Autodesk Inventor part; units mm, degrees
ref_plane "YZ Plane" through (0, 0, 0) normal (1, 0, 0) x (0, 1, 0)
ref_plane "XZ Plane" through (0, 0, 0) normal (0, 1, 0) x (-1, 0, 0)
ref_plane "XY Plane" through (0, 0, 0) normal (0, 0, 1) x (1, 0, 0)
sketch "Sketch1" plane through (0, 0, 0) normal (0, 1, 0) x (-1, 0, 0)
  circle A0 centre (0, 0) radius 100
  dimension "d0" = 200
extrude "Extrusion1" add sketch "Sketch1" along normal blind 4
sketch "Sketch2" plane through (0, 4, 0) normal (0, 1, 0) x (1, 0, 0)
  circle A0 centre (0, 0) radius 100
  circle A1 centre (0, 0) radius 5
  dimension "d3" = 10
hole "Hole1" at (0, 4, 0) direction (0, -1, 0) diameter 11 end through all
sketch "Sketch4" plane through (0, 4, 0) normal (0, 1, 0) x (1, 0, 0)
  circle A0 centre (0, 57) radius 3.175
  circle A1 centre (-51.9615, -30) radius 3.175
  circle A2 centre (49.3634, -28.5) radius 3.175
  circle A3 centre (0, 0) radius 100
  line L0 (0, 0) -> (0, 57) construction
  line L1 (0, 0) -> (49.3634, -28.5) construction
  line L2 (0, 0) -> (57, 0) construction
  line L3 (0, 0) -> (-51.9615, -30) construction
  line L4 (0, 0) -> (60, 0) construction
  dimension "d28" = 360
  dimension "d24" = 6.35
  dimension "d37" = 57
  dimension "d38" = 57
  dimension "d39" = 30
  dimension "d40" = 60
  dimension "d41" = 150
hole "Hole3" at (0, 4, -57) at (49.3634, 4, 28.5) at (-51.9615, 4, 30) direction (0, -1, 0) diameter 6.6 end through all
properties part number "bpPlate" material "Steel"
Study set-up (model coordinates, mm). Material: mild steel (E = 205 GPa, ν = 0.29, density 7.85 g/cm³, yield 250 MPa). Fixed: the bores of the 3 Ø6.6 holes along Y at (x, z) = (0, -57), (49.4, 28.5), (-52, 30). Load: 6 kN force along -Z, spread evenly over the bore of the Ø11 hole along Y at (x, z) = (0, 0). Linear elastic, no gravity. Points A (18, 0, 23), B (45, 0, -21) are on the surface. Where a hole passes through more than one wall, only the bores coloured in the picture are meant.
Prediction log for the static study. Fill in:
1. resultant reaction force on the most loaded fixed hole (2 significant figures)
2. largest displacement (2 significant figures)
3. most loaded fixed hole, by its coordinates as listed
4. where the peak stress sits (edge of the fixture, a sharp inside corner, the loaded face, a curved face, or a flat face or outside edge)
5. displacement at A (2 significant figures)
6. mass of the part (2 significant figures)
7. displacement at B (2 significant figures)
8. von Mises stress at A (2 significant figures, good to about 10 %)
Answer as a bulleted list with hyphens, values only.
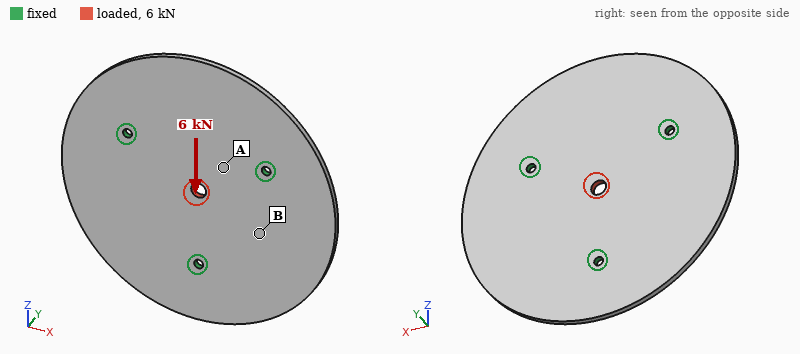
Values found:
- 2.3 kN
- 6.4 µm
- (0, -57)
- the loaded face
- 3.1 µm
- 980 g
- 1.7 µm
- 12 MPa
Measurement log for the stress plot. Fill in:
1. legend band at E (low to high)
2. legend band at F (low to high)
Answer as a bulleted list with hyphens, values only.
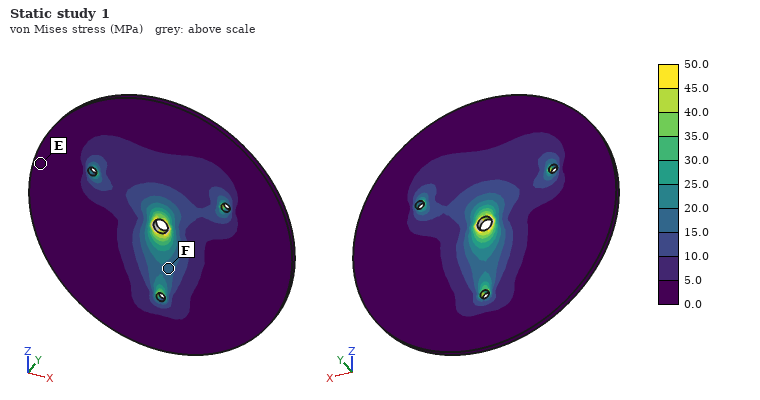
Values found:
- 0.0 to 5.0 MPa
- 15.0 to 20.0 MPa
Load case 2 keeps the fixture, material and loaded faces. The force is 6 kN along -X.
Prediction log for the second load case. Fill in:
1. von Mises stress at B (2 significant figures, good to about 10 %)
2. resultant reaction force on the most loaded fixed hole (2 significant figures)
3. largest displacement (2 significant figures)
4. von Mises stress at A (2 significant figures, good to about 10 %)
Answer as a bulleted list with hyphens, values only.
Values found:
- 5.7 MPa
- 2.2 kN
- 6.4 µm
- 13 MPa
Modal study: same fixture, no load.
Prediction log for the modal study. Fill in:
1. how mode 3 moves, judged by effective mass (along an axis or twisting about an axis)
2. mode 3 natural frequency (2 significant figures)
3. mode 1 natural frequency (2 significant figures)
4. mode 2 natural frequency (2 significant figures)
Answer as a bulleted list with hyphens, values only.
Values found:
- along Y
- 810 Hz
- 670 Hz
- 680 Hz
